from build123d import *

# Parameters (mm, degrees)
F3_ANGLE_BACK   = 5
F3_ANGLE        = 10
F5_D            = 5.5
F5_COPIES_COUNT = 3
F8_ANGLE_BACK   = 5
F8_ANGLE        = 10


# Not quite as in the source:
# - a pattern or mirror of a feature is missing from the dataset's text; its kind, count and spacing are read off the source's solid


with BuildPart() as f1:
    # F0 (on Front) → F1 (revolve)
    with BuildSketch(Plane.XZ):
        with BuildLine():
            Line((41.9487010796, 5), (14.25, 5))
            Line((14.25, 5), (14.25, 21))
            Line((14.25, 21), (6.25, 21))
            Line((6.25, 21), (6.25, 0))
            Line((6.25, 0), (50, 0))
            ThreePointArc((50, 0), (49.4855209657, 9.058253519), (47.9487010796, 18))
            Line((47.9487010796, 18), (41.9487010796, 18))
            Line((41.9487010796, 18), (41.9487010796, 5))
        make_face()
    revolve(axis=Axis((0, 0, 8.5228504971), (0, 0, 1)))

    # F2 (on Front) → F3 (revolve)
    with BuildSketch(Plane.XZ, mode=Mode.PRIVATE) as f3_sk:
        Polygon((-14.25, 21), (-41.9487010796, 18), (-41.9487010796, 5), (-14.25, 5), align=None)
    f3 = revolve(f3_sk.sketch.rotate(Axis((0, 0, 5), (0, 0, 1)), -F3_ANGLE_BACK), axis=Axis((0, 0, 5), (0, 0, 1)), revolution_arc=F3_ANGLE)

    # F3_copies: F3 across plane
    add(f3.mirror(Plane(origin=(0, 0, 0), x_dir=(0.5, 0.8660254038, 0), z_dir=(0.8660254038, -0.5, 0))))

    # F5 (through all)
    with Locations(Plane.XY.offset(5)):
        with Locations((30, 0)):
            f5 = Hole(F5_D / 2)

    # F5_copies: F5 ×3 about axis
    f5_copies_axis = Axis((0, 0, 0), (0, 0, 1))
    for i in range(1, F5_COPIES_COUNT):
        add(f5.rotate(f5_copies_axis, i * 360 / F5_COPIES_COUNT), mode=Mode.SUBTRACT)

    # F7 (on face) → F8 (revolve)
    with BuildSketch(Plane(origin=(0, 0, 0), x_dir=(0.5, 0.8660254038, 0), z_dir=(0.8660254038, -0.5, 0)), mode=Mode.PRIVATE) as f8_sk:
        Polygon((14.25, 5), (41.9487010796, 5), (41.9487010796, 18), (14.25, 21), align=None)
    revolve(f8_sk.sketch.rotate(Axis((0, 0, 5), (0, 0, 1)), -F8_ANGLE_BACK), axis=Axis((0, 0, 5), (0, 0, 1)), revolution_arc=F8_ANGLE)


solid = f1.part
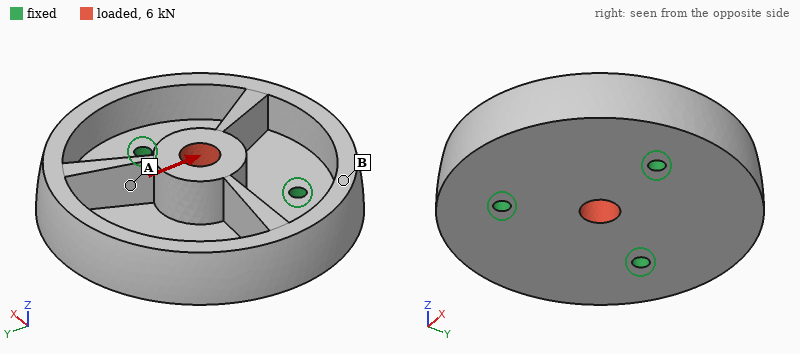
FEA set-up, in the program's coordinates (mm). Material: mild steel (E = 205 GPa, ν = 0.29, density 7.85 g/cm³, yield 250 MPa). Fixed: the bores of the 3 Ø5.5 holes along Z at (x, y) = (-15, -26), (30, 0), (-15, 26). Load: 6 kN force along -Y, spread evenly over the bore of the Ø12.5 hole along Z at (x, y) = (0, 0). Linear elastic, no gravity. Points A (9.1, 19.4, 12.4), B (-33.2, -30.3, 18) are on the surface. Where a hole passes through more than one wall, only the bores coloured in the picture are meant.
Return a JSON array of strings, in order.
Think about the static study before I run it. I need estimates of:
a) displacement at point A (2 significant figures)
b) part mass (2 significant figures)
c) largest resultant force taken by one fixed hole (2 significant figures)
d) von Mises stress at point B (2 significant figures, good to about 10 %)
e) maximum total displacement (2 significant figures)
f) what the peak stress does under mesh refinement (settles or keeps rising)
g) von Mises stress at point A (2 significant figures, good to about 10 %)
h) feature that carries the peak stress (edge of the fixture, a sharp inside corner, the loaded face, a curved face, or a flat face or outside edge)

["6.7 µm", "620 g", "2.2 kN", "7.4 MPa", "11 µm", "keeps rising", "19 MPa", "edge of the fixture"]
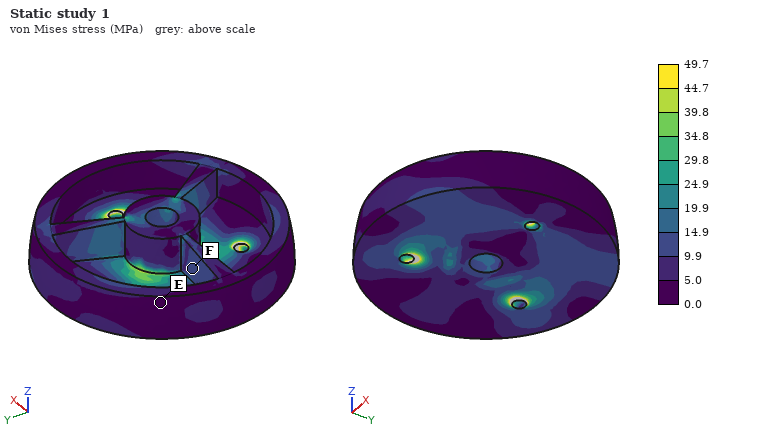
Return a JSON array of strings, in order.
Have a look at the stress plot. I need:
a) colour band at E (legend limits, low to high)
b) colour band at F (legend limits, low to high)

["0.0 to 5.0 MPa", "9.9 to 14.9 MPa"]
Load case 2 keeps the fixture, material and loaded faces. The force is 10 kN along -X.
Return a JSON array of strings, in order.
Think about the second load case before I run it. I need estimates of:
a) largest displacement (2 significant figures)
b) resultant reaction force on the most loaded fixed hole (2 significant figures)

["20 µm", "3.8 kN"]
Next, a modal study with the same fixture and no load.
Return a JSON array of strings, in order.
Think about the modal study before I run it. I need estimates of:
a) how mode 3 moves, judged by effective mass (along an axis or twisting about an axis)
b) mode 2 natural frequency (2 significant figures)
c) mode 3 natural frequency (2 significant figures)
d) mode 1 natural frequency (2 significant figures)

["along Z", "4100 Hz", "5900 Hz", "4100 Hz"]
